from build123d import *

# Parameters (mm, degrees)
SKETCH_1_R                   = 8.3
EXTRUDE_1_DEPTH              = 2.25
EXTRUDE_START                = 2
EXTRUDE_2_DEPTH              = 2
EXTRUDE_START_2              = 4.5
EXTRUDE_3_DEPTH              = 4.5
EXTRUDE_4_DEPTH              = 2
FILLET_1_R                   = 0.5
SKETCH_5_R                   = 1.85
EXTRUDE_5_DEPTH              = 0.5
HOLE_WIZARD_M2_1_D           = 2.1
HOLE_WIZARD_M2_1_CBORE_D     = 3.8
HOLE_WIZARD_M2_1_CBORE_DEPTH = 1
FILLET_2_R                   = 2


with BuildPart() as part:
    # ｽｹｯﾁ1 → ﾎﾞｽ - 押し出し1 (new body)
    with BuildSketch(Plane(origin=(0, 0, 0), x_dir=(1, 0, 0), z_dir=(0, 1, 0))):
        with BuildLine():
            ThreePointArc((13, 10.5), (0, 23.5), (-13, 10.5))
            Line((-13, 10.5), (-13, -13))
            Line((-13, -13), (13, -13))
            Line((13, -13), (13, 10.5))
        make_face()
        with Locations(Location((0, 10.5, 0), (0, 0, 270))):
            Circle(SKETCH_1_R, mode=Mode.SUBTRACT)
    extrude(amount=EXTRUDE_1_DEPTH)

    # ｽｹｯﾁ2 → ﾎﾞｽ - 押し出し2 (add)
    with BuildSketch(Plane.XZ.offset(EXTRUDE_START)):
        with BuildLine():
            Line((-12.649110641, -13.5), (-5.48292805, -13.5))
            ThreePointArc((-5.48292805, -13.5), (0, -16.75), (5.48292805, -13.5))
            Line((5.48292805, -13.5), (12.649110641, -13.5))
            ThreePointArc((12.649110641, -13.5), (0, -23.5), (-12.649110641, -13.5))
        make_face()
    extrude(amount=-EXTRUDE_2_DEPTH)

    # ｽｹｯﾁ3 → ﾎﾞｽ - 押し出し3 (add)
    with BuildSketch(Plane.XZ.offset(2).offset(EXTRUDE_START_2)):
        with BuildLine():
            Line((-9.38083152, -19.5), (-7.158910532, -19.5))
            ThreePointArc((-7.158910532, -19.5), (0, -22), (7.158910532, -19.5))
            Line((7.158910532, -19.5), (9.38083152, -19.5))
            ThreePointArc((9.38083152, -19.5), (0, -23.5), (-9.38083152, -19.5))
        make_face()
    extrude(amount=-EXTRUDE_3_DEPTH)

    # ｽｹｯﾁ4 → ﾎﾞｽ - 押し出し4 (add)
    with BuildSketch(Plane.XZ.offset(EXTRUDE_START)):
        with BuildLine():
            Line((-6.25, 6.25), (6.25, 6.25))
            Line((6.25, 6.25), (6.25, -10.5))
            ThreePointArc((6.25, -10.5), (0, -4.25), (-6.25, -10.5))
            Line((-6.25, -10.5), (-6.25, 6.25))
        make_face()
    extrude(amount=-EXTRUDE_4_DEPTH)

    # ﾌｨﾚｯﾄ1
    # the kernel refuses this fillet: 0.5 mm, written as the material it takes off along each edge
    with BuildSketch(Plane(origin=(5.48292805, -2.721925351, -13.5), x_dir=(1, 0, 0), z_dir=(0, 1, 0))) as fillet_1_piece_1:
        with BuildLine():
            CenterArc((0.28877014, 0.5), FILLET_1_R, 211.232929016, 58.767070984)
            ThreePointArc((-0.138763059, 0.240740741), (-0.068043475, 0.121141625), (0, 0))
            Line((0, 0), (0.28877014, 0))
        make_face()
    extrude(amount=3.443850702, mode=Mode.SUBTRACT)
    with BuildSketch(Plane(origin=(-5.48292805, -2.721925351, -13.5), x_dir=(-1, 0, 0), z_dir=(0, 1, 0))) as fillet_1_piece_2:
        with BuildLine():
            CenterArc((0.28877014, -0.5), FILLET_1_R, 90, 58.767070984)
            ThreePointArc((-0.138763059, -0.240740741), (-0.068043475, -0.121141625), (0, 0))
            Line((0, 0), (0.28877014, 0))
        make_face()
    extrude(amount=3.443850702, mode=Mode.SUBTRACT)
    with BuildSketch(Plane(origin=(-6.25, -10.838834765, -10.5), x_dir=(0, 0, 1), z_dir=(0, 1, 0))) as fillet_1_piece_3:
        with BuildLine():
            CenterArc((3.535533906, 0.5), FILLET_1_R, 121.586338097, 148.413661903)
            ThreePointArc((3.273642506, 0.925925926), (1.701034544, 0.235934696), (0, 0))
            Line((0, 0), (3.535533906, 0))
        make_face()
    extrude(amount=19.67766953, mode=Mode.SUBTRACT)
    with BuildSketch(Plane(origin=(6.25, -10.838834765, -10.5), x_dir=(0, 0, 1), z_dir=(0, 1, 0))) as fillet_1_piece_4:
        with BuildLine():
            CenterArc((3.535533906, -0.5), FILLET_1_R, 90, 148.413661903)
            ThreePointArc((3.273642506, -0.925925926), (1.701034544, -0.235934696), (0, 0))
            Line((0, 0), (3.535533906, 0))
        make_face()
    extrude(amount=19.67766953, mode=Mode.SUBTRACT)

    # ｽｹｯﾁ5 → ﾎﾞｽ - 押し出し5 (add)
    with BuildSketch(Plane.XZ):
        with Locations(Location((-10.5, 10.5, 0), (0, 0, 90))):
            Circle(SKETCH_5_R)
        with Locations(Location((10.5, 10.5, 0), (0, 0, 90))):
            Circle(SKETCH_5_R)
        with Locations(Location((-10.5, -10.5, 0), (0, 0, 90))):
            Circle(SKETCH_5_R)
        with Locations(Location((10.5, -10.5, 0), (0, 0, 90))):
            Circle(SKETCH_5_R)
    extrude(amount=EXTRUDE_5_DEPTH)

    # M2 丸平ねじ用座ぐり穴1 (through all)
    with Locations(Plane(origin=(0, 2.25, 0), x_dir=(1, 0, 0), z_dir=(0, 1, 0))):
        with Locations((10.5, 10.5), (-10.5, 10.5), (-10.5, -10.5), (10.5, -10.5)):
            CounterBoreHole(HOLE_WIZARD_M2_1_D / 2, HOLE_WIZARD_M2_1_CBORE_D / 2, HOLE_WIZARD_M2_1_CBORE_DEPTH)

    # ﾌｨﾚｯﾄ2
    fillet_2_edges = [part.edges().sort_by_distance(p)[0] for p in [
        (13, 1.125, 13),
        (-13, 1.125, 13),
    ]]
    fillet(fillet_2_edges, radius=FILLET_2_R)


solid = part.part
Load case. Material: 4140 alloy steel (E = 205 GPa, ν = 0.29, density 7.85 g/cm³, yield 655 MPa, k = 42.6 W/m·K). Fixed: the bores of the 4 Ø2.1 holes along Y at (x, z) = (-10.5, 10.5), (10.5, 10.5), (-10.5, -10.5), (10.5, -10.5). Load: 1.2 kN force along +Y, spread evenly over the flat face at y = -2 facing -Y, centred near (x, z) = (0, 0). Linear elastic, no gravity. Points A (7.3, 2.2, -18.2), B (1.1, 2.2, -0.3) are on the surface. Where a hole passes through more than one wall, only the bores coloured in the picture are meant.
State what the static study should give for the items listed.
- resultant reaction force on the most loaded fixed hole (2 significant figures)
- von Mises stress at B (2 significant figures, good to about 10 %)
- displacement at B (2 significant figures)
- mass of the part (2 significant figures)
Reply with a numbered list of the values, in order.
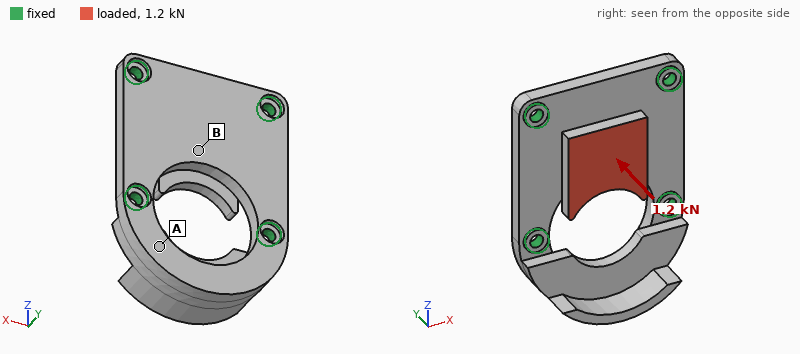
1. 410 N
2. 96 MPa
3. 25 µm
4. 17 g
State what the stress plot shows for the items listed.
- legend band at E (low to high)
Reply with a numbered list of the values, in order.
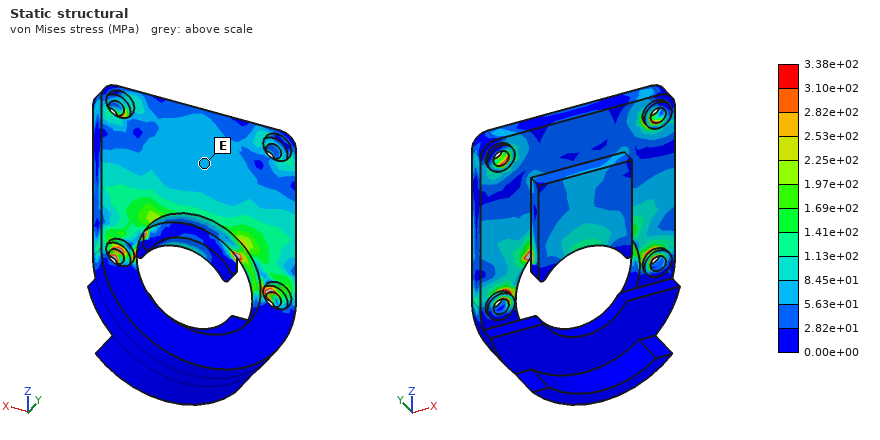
1. 5.63e+01 to 8.45e+01 MPa
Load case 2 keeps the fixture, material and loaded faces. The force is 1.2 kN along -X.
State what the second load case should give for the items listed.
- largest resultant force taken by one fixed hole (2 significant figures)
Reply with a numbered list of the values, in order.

1. 500 N
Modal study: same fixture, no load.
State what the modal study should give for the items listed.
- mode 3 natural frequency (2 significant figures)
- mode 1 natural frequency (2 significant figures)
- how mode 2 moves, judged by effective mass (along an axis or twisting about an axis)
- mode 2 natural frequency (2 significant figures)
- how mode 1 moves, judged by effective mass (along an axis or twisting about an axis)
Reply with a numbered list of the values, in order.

1. 21 kHz
2. 4900 Hz
3. along Y
4. 15 kHz
5. along Y
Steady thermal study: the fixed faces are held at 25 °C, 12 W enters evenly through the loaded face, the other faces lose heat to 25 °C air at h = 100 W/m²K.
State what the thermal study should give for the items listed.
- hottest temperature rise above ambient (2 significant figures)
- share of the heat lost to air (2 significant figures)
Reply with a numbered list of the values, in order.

1. 46 K
2. 23 %
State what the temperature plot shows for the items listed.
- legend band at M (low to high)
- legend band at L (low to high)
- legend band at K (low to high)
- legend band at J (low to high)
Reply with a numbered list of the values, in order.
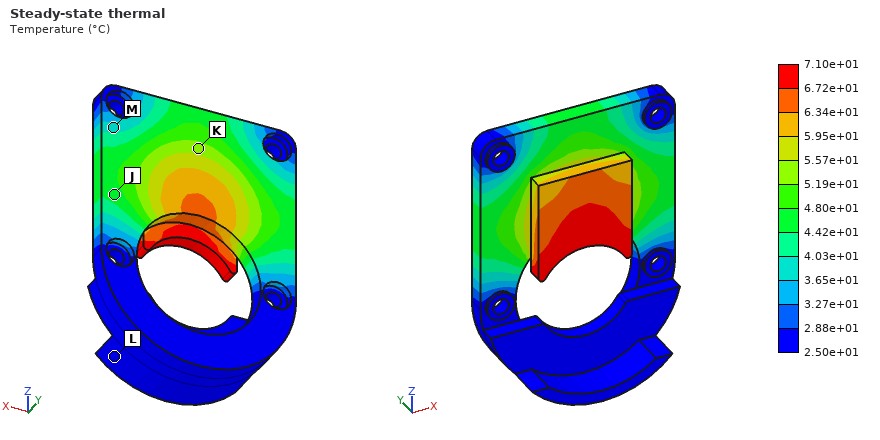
1. 3.65e+01 to 4.03e+01 °C
2. 2.50e+01 to 2.88e+01 °C
3. 5.19e+01 to 5.57e+01 °C
4. 4.42e+01 to 4.80e+01 °C
